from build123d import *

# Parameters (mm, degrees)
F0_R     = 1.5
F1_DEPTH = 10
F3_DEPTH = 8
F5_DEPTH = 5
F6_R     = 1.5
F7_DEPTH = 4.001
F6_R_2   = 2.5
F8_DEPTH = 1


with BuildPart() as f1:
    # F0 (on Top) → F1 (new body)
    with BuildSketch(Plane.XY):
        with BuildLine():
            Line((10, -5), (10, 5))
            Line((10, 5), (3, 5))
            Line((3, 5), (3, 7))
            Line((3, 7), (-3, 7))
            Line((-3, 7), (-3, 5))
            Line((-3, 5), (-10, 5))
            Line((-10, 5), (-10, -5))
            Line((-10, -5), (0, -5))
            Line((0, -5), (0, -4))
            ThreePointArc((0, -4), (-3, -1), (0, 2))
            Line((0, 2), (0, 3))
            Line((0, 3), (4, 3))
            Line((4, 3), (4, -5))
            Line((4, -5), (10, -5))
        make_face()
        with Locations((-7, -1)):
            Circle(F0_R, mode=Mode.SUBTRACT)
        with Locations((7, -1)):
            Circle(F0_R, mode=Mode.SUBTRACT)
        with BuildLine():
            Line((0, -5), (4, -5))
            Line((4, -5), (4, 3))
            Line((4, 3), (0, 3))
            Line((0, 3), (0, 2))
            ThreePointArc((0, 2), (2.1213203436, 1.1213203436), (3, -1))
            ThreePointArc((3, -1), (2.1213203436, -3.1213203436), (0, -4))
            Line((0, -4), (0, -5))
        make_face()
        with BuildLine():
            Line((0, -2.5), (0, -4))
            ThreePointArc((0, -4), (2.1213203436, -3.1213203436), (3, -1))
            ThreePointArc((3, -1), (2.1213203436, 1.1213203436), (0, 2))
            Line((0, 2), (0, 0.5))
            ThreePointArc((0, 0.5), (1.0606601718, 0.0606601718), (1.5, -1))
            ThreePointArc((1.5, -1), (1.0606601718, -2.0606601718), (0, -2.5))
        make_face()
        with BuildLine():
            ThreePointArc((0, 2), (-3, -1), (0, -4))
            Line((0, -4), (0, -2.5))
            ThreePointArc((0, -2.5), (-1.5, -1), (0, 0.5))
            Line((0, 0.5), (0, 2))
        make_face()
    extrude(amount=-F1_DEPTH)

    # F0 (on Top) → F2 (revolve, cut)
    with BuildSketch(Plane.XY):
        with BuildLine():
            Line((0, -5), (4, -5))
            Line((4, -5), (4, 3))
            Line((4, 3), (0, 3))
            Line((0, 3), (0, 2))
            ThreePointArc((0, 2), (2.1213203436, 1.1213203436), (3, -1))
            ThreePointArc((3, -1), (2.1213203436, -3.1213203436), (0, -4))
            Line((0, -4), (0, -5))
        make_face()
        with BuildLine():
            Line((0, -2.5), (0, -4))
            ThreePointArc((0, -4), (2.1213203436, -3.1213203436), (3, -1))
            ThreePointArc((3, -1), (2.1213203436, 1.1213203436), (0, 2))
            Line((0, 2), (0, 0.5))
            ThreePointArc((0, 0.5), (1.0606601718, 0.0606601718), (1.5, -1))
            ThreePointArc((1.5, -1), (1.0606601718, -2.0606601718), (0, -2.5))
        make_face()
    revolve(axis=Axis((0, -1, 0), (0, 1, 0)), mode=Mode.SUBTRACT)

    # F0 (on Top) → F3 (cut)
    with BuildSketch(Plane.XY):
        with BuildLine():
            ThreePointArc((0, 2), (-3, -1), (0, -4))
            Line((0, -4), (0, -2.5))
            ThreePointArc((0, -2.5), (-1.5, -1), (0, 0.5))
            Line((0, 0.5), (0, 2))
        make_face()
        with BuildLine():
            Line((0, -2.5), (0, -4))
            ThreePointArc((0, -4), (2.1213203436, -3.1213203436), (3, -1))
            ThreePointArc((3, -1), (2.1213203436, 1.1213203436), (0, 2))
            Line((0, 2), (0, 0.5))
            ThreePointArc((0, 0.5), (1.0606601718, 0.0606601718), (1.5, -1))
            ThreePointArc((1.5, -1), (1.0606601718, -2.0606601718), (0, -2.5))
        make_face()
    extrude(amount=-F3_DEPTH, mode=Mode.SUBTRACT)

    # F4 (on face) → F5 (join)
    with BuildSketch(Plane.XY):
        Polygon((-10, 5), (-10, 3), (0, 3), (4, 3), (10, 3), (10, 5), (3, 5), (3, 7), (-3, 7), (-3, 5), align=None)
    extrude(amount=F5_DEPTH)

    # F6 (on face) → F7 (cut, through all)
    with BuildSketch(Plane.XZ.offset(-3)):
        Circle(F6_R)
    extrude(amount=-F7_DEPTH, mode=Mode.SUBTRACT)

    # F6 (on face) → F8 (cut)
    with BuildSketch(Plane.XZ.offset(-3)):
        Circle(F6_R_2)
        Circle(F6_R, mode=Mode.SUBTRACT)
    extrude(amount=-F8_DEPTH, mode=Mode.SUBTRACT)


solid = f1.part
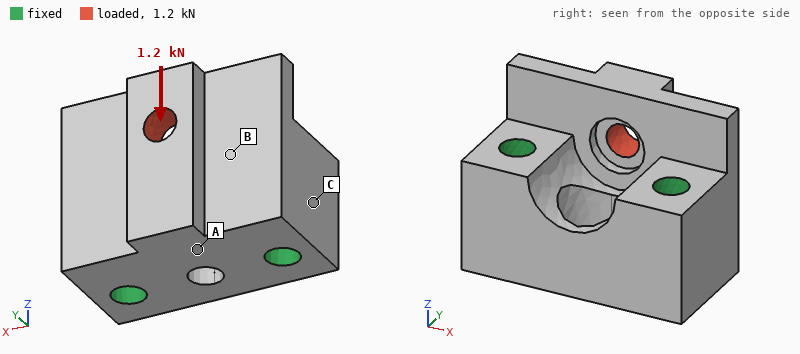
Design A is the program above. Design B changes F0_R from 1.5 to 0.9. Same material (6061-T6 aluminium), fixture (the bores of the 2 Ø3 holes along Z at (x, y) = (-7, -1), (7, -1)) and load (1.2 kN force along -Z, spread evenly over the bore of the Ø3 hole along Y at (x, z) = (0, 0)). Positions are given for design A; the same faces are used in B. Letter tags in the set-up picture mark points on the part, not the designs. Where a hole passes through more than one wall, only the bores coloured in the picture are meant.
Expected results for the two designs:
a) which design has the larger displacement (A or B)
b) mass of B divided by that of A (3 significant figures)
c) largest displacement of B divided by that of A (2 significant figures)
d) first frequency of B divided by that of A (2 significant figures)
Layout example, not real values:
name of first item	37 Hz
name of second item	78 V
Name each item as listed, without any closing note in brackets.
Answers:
which design has the larger displacement	B
mass of B divided by that of A	1.05
largest displacement of B divided by that of A	1.1
first frequency of B divided by that of A	0.97
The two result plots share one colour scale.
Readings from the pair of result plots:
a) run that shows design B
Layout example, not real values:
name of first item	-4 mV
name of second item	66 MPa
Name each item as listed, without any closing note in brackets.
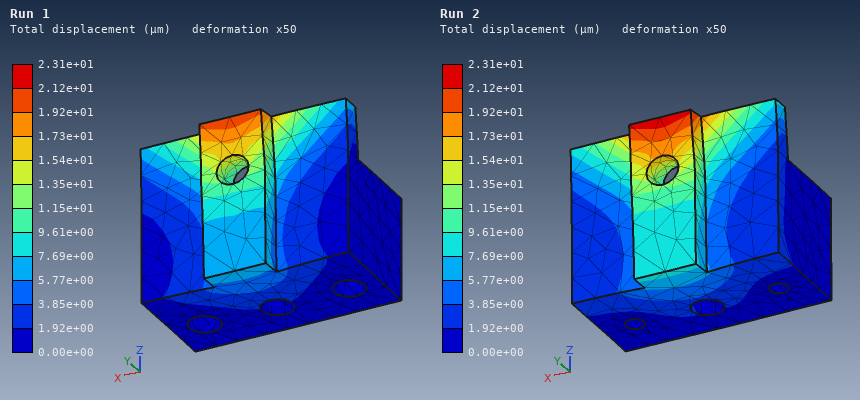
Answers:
run that shows design B	Run 2
